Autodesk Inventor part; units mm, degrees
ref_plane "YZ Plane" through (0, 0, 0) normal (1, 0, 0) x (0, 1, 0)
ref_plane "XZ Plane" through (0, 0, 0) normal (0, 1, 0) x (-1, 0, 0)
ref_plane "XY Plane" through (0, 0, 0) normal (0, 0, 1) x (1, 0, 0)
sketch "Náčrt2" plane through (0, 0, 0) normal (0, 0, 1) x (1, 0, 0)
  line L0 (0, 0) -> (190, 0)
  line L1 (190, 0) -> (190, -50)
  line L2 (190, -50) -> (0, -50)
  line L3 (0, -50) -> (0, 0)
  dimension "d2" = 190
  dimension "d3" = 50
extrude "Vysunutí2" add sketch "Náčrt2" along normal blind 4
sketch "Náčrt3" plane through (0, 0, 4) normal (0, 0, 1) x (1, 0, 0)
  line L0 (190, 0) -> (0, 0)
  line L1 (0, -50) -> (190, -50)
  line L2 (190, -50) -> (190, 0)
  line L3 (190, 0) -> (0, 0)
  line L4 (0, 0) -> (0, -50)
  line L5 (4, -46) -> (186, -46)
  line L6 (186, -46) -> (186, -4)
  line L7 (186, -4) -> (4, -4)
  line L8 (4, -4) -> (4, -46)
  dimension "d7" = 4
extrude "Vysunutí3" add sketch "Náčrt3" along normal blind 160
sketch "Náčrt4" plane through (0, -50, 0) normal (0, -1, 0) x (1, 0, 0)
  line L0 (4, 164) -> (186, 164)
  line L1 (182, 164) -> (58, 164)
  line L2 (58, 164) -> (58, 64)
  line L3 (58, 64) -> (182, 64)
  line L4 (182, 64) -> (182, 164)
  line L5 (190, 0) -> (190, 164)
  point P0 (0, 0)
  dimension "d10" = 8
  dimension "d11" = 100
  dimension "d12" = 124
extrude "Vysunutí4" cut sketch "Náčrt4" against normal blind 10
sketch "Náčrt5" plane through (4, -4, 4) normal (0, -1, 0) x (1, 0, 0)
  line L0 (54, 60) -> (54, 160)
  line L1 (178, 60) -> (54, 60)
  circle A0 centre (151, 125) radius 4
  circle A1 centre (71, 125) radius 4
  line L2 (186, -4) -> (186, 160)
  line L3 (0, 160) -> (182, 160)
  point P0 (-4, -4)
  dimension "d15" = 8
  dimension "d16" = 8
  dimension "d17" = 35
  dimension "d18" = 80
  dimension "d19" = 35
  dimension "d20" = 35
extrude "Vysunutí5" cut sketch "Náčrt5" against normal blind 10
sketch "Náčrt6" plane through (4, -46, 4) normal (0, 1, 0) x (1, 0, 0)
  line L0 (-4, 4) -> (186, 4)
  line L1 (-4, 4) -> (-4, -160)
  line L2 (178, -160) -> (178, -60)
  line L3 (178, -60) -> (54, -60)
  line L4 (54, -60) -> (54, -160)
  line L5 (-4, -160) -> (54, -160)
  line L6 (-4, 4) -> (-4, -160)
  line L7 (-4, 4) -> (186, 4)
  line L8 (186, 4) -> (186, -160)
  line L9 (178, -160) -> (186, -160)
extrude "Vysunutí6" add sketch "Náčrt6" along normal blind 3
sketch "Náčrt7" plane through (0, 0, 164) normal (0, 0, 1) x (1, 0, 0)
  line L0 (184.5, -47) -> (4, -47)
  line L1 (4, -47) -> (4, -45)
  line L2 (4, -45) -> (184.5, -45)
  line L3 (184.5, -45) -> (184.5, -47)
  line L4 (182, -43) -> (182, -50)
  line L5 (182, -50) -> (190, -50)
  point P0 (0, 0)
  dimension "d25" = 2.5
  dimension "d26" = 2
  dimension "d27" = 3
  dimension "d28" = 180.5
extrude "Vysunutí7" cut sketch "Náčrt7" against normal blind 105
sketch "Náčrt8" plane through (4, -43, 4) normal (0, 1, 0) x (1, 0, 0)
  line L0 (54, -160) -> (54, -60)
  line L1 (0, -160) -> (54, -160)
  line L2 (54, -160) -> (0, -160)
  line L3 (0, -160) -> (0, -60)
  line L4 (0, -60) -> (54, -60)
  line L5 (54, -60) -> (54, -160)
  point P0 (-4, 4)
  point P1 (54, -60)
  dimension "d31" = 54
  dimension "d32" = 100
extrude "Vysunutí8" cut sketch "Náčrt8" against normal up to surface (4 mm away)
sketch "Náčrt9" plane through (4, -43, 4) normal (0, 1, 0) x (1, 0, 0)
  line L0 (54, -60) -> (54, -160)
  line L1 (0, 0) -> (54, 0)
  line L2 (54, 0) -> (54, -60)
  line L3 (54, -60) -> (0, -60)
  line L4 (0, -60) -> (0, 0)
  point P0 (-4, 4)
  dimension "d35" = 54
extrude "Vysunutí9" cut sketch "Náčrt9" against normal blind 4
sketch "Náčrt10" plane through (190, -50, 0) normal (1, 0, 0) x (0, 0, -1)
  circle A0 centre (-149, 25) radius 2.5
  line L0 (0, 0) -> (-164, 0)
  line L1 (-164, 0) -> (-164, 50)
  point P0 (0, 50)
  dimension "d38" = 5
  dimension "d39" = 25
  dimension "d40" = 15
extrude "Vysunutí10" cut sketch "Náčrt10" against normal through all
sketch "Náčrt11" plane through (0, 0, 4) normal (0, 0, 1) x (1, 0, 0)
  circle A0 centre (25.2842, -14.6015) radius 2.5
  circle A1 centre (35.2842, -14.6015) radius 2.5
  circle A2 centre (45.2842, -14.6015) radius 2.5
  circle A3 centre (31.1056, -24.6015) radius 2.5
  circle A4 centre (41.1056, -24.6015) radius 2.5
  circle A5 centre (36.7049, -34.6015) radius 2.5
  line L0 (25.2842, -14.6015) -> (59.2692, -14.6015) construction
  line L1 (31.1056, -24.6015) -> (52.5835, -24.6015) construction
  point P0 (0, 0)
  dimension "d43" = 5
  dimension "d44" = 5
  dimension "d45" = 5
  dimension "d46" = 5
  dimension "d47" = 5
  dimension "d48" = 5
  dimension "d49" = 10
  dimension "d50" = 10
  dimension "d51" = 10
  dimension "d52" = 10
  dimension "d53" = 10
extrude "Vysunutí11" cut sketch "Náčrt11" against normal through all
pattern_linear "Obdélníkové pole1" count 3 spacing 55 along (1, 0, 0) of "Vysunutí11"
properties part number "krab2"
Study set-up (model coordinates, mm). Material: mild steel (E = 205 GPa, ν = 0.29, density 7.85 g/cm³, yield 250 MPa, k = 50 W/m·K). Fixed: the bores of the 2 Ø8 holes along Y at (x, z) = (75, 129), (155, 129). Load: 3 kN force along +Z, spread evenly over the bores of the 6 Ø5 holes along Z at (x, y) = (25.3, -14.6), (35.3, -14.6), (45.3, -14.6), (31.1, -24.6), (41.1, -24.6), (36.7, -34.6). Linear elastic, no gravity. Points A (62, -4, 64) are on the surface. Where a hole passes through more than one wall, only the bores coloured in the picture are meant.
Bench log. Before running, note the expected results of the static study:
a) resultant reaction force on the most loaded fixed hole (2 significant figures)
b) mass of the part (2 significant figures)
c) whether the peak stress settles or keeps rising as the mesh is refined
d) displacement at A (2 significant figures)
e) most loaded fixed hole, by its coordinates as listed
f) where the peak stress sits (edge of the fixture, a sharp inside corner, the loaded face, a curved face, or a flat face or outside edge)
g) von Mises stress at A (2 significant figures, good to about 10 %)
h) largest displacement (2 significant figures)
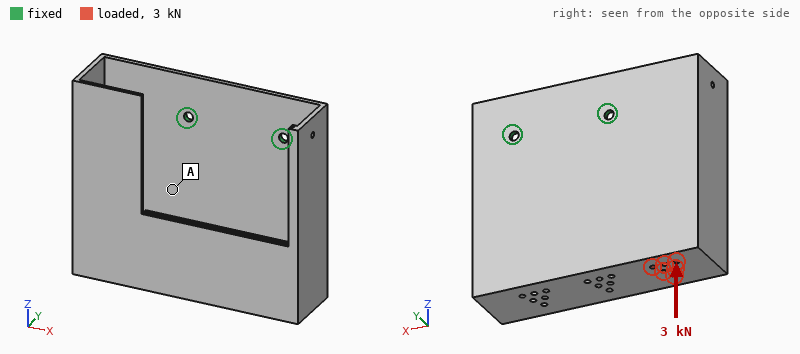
4.4 kN
2.3 kg
keeps rising
0.35 mm
(75, 129)
edge of the fixture
20 MPa
1.0 mm
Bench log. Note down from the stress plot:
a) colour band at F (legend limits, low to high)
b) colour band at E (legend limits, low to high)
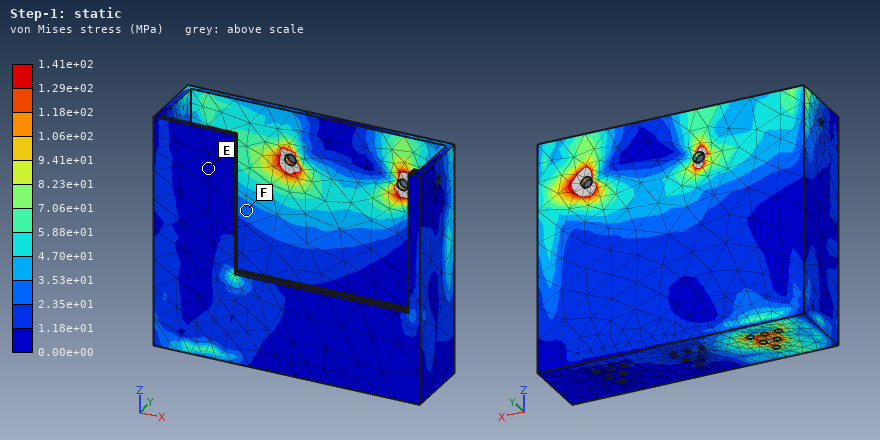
2.35e+01 to 3.53e+01 MPa
0.00e+00 to 1.18e+01 MPa
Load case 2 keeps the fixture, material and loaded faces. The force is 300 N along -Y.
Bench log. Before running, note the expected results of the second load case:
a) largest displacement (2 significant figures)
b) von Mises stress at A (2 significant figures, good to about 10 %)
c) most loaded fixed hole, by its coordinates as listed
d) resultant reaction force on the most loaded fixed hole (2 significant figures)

0.78 mm
13 MPa
(75, 129)
330 N
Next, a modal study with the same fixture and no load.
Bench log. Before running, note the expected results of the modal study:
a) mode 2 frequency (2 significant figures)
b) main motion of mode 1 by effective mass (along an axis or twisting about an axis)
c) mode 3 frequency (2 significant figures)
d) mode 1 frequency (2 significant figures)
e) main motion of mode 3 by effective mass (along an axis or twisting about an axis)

200 Hz
along Y
450 Hz
120 Hz
along Y
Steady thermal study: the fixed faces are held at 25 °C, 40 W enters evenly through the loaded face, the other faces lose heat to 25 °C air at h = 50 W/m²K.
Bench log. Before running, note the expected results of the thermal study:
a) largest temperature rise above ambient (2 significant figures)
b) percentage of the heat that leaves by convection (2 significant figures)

68 K
98 %
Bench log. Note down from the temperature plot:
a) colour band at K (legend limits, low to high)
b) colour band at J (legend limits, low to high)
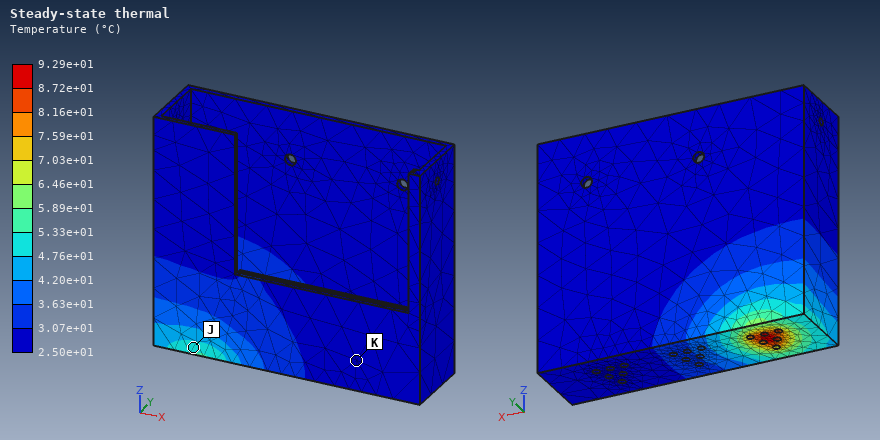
2.50e+01 to 3.07e+01 °C
4.76e+01 to 5.33e+01 °C
